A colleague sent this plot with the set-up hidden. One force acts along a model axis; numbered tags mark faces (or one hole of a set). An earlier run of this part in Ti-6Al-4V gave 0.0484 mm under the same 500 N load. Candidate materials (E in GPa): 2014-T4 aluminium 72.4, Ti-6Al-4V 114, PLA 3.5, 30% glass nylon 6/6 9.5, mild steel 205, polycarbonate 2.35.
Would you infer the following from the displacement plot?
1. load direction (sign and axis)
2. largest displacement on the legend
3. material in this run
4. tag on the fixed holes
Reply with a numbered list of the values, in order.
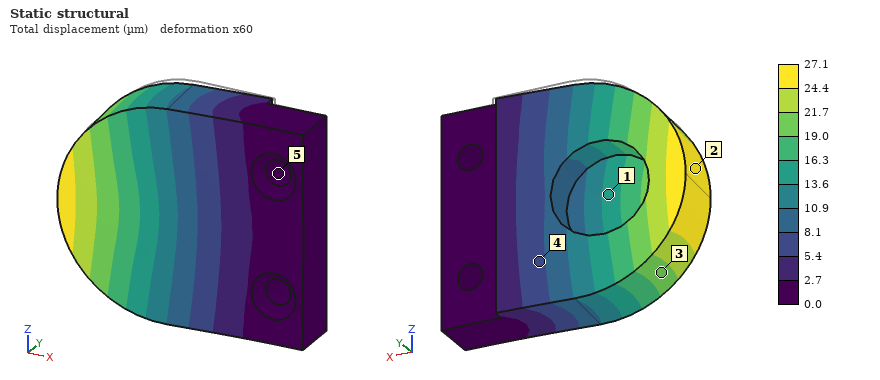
1. -Y
2. 27.1 µm
3. mild steel
4. 5
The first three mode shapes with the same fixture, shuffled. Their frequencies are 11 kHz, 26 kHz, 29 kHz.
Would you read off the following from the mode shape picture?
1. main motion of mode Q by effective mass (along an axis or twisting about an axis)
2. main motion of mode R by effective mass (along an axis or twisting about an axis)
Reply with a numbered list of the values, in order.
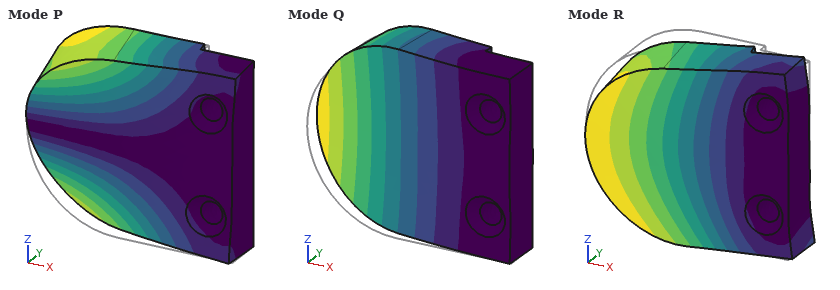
1. along Y
2. along Z
